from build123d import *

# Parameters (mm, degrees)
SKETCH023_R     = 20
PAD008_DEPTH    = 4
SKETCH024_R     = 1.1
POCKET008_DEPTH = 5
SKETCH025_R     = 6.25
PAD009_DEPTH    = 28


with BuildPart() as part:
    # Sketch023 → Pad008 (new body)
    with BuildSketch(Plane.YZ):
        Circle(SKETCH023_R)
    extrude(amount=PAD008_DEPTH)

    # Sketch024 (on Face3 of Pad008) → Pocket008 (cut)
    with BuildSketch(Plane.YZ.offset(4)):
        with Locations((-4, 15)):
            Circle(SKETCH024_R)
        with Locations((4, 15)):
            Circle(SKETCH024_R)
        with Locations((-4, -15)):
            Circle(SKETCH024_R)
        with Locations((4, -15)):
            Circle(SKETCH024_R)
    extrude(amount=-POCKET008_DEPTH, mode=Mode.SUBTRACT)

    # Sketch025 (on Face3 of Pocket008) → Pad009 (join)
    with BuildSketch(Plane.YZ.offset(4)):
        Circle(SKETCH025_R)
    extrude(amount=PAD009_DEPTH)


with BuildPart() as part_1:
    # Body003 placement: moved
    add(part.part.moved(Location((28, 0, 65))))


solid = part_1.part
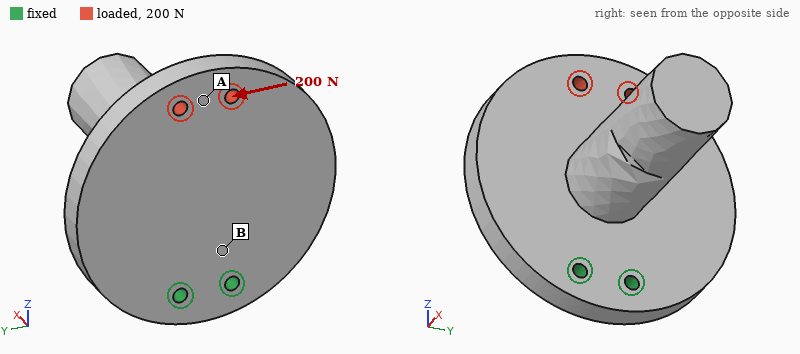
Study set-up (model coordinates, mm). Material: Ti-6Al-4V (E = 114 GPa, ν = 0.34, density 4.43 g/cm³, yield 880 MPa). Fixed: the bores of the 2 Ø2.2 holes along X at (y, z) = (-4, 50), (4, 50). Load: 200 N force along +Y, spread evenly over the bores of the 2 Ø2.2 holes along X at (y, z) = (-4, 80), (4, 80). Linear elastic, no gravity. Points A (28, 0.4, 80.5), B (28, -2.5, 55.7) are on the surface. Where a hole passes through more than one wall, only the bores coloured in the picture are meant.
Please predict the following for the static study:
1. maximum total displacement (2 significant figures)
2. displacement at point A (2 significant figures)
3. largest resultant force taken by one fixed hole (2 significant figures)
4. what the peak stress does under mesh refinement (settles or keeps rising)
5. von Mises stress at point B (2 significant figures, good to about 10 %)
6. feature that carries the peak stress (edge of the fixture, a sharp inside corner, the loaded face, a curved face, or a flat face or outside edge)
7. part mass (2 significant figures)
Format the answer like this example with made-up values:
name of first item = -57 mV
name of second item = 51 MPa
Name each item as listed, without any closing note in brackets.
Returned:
maximum total displacement = 12 µm
displacement at point A = 10 µm
largest resultant force taken by one fixed hole = 610 N
what the peak stress does under mesh refinement = keeps rising
von Mises stress at point B = 15 MPa
feature that carries the peak stress = edge of the fixture
part mass = 37 g
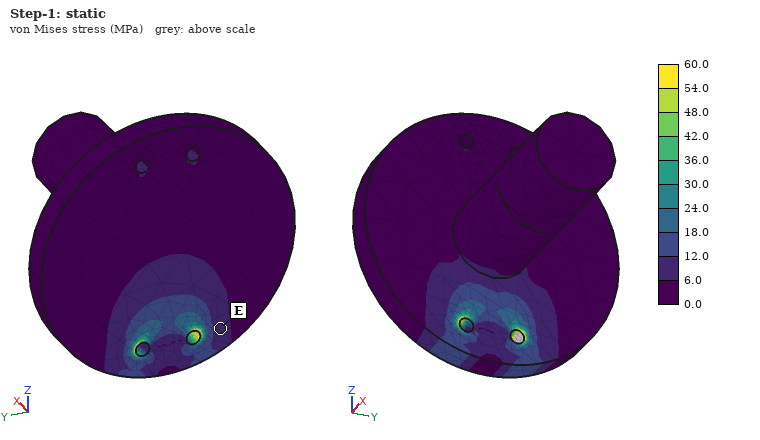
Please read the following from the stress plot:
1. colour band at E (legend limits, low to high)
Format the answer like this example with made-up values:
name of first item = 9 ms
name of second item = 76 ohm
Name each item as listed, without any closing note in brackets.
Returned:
colour band at E = 6.0 to 12.0 MPa
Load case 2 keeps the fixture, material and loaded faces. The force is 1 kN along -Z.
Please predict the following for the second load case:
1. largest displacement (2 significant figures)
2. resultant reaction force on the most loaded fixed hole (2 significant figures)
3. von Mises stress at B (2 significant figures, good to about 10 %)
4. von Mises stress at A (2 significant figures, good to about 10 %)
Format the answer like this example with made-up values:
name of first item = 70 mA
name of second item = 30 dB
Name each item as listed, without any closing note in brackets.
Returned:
largest displacement = 4.2 µm
resultant reaction force on the most loaded fixed hole = 500 N
von Mises stress at B = 14 MPa
von Mises stress at A = 6.7 MPa
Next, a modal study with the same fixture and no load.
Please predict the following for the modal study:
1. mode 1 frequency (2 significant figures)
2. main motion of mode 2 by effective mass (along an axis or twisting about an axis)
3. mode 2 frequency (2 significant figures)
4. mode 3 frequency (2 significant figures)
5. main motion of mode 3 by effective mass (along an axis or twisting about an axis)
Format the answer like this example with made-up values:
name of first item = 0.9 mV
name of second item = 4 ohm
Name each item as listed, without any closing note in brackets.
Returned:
mode 1 frequency = 1700 Hz
main motion of mode 2 by effective mass = along Y
mode 2 frequency = 3100 Hz
mode 3 frequency = 6600 Hz
main motion of mode 3 by effective mass = along Y
